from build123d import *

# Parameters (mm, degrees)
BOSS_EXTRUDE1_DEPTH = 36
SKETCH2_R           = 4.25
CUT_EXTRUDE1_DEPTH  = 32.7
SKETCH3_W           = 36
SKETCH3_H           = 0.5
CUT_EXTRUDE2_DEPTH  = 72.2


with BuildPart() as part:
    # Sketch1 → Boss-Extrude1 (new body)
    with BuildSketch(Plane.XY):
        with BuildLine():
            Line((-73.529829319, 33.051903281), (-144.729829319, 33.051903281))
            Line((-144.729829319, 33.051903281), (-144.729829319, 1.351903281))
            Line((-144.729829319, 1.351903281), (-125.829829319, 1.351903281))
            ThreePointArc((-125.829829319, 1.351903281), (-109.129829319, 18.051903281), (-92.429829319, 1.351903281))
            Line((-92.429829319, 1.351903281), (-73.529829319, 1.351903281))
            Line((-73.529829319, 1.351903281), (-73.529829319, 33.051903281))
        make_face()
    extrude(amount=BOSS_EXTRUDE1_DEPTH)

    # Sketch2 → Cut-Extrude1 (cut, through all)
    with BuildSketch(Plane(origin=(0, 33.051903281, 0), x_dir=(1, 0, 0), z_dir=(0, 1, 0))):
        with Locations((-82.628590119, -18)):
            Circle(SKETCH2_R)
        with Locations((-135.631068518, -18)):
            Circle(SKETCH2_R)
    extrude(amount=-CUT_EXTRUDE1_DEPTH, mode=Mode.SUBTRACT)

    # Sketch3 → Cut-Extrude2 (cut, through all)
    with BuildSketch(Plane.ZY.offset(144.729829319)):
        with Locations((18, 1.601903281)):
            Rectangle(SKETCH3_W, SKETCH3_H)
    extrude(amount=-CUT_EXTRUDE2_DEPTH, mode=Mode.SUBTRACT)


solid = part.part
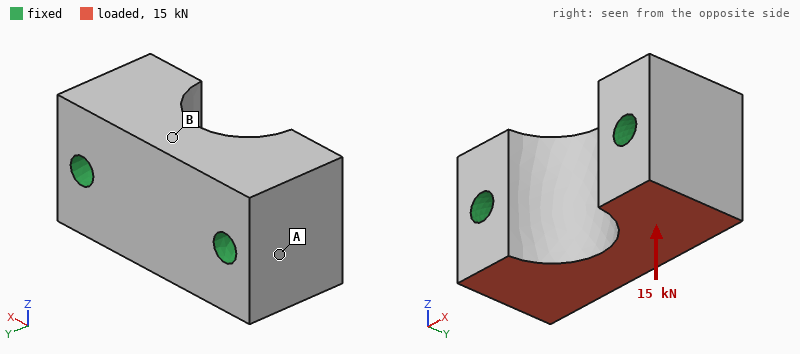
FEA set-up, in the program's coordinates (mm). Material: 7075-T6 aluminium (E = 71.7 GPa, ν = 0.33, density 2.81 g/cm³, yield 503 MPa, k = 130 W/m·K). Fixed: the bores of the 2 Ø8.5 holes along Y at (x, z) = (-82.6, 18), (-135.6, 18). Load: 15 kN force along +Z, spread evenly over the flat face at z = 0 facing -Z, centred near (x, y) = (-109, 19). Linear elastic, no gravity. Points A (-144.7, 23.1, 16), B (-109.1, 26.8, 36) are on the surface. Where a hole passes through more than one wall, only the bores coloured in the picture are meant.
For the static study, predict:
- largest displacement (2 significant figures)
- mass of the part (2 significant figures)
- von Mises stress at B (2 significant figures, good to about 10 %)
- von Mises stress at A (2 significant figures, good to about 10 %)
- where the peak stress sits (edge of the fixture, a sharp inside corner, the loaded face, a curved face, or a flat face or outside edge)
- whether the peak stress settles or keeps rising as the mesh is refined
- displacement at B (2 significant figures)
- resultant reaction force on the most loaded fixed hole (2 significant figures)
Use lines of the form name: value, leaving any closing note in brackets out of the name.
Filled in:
largest displacement: 6.5 µm
mass of the part: 170 g
von Mises stress at B: 8.6 MPa
von Mises stress at A: 4.1 MPa
where the peak stress sits: edge of the fixture
whether the peak stress settles or keeps rising as the mesh is refined: keeps rising
displacement at B: 3.7 µm
resultant reaction force on the most loaded fixed hole: 7.5 kN
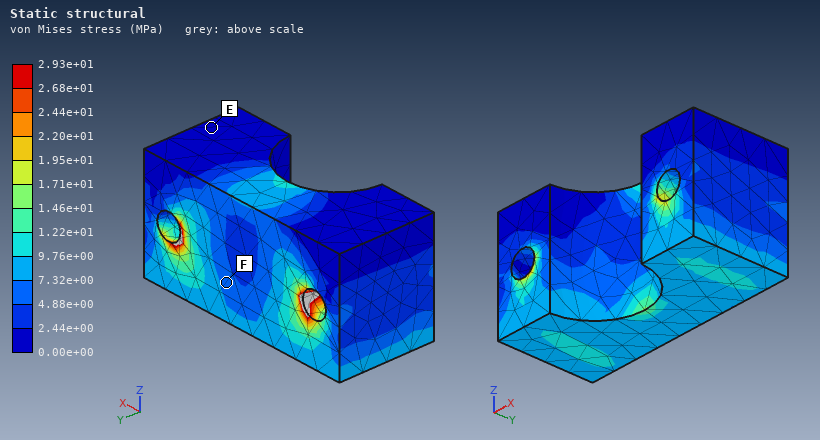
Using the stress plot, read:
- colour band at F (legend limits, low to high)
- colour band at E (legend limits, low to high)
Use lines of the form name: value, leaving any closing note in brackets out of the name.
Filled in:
colour band at F: 4.88e+00 to 7.32e+00 MPa
colour band at E: 0.00e+00 to 2.44e+00 MPa
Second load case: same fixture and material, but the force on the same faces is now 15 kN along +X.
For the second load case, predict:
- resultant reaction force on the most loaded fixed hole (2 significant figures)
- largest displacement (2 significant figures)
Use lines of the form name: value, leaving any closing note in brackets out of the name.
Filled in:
resultant reaction force on the most loaded fixed hole: 8.3 kN
largest displacement: 13 µm
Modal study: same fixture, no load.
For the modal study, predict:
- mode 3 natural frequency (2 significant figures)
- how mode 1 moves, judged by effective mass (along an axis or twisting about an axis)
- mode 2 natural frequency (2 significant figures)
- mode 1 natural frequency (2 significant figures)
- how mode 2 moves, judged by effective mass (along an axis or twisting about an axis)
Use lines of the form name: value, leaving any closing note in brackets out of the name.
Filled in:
mode 3 natural frequency: 30 kHz
how mode 1 moves, judged by effective mass: along Z
mode 2 natural frequency: 25 kHz
mode 1 natural frequency: 22 kHz
how mode 2 moves, judged by effective mass: along Y
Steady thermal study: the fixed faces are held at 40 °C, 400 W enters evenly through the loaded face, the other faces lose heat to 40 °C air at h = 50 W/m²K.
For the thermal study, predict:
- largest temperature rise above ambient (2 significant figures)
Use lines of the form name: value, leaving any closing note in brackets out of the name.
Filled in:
largest temperature rise above ambient: 39 K
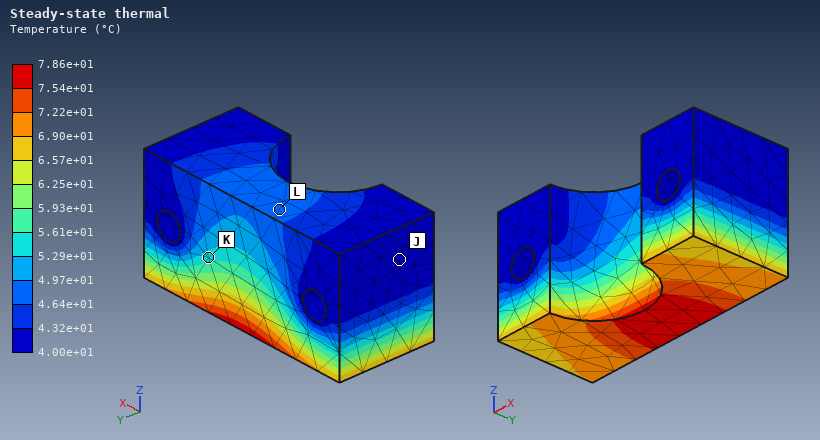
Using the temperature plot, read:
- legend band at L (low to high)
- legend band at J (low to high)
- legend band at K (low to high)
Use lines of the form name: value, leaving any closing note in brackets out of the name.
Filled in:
legend band at L: 4.64e+01 to 4.97e+01 °C
legend band at J: 4.00e+01 to 4.32e+01 °C
legend band at K: 5.29e+01 to 5.61e+01 °C
